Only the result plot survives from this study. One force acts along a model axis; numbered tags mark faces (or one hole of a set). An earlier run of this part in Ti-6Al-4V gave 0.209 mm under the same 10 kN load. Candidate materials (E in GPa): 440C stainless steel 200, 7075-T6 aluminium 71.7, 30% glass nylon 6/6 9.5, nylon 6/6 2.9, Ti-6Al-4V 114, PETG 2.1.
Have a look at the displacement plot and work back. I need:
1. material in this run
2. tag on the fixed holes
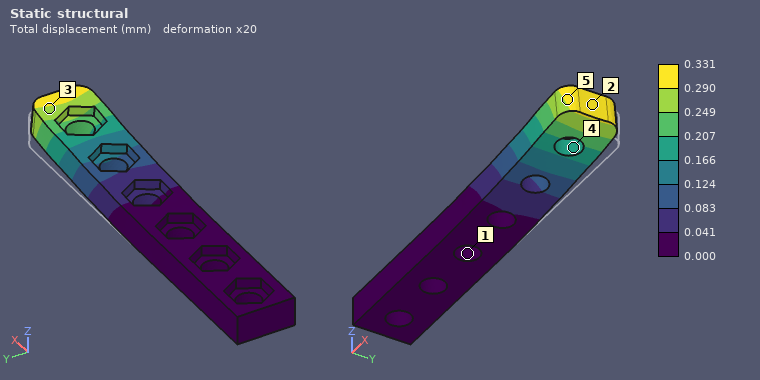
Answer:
7075-T6 aluminium
1
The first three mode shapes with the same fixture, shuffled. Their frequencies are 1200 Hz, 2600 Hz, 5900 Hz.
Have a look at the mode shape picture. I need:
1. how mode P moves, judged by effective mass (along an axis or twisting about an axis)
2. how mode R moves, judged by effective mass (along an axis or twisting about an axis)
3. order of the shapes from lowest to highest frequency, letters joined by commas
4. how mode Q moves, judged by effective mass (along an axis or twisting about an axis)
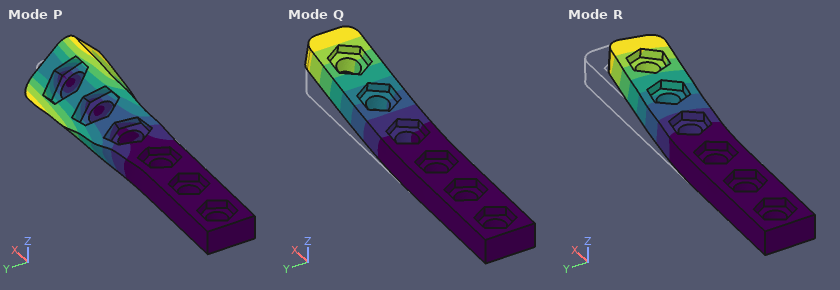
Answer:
twisting about X
along Y
Q, R, P
along Z
